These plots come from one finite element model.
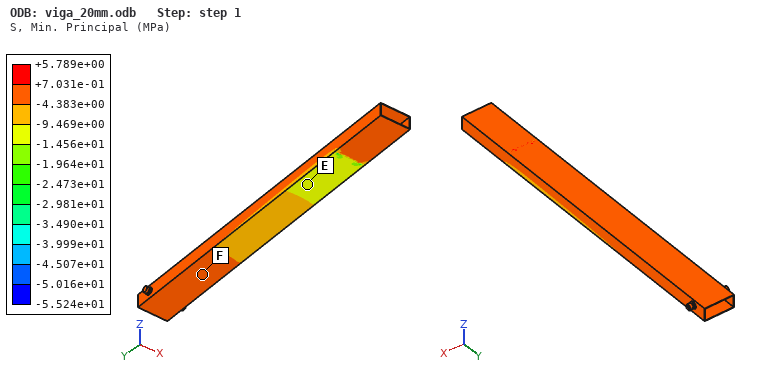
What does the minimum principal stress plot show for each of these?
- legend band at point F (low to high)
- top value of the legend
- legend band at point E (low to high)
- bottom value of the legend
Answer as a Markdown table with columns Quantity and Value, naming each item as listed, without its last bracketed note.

| Quantity | Value |
|---|---|
| legend band at point F | -4.383e+00 to +7.031e-01 MPa |
| top value of the legend | +5.789e+00 MPa |
| legend band at point E | -1.456e+01 to -9.469e+00 MPa |
| bottom value of the legend | -5.524e+01 MPa |
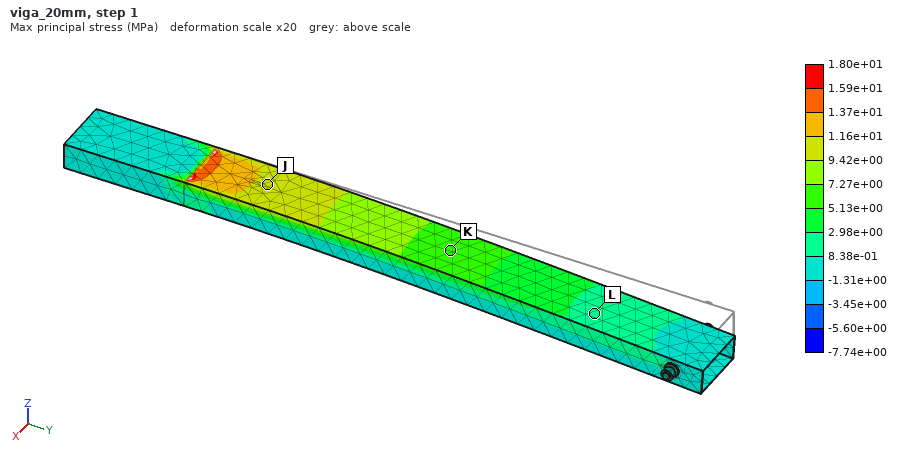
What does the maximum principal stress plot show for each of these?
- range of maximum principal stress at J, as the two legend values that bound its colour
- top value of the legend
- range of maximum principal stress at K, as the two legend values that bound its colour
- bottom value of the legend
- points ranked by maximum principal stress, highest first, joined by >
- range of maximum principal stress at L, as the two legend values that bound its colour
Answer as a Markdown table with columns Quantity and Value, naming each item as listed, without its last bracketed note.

| Quantity | Value |
|---|---|
| range of maximum principal stress at J, as the two legend values that bound its colour | 9.42e+00 to 1.16e+01 MPa |
| top value of the legend | 1.80e+01 MPa |
| range of maximum principal stress at K, as the two legend values that bound its colour | 5.13e+00 to 7.27e+00 MPa |
| bottom value of the legend | -7.74e+00 MPa |
| points ranked by maximum principal stress, highest first, joined by > | J > K > L |
| range of maximum principal stress at L, as the two legend values that bound its colour | 8.38e-01 to 2.98e+00 MPa |
